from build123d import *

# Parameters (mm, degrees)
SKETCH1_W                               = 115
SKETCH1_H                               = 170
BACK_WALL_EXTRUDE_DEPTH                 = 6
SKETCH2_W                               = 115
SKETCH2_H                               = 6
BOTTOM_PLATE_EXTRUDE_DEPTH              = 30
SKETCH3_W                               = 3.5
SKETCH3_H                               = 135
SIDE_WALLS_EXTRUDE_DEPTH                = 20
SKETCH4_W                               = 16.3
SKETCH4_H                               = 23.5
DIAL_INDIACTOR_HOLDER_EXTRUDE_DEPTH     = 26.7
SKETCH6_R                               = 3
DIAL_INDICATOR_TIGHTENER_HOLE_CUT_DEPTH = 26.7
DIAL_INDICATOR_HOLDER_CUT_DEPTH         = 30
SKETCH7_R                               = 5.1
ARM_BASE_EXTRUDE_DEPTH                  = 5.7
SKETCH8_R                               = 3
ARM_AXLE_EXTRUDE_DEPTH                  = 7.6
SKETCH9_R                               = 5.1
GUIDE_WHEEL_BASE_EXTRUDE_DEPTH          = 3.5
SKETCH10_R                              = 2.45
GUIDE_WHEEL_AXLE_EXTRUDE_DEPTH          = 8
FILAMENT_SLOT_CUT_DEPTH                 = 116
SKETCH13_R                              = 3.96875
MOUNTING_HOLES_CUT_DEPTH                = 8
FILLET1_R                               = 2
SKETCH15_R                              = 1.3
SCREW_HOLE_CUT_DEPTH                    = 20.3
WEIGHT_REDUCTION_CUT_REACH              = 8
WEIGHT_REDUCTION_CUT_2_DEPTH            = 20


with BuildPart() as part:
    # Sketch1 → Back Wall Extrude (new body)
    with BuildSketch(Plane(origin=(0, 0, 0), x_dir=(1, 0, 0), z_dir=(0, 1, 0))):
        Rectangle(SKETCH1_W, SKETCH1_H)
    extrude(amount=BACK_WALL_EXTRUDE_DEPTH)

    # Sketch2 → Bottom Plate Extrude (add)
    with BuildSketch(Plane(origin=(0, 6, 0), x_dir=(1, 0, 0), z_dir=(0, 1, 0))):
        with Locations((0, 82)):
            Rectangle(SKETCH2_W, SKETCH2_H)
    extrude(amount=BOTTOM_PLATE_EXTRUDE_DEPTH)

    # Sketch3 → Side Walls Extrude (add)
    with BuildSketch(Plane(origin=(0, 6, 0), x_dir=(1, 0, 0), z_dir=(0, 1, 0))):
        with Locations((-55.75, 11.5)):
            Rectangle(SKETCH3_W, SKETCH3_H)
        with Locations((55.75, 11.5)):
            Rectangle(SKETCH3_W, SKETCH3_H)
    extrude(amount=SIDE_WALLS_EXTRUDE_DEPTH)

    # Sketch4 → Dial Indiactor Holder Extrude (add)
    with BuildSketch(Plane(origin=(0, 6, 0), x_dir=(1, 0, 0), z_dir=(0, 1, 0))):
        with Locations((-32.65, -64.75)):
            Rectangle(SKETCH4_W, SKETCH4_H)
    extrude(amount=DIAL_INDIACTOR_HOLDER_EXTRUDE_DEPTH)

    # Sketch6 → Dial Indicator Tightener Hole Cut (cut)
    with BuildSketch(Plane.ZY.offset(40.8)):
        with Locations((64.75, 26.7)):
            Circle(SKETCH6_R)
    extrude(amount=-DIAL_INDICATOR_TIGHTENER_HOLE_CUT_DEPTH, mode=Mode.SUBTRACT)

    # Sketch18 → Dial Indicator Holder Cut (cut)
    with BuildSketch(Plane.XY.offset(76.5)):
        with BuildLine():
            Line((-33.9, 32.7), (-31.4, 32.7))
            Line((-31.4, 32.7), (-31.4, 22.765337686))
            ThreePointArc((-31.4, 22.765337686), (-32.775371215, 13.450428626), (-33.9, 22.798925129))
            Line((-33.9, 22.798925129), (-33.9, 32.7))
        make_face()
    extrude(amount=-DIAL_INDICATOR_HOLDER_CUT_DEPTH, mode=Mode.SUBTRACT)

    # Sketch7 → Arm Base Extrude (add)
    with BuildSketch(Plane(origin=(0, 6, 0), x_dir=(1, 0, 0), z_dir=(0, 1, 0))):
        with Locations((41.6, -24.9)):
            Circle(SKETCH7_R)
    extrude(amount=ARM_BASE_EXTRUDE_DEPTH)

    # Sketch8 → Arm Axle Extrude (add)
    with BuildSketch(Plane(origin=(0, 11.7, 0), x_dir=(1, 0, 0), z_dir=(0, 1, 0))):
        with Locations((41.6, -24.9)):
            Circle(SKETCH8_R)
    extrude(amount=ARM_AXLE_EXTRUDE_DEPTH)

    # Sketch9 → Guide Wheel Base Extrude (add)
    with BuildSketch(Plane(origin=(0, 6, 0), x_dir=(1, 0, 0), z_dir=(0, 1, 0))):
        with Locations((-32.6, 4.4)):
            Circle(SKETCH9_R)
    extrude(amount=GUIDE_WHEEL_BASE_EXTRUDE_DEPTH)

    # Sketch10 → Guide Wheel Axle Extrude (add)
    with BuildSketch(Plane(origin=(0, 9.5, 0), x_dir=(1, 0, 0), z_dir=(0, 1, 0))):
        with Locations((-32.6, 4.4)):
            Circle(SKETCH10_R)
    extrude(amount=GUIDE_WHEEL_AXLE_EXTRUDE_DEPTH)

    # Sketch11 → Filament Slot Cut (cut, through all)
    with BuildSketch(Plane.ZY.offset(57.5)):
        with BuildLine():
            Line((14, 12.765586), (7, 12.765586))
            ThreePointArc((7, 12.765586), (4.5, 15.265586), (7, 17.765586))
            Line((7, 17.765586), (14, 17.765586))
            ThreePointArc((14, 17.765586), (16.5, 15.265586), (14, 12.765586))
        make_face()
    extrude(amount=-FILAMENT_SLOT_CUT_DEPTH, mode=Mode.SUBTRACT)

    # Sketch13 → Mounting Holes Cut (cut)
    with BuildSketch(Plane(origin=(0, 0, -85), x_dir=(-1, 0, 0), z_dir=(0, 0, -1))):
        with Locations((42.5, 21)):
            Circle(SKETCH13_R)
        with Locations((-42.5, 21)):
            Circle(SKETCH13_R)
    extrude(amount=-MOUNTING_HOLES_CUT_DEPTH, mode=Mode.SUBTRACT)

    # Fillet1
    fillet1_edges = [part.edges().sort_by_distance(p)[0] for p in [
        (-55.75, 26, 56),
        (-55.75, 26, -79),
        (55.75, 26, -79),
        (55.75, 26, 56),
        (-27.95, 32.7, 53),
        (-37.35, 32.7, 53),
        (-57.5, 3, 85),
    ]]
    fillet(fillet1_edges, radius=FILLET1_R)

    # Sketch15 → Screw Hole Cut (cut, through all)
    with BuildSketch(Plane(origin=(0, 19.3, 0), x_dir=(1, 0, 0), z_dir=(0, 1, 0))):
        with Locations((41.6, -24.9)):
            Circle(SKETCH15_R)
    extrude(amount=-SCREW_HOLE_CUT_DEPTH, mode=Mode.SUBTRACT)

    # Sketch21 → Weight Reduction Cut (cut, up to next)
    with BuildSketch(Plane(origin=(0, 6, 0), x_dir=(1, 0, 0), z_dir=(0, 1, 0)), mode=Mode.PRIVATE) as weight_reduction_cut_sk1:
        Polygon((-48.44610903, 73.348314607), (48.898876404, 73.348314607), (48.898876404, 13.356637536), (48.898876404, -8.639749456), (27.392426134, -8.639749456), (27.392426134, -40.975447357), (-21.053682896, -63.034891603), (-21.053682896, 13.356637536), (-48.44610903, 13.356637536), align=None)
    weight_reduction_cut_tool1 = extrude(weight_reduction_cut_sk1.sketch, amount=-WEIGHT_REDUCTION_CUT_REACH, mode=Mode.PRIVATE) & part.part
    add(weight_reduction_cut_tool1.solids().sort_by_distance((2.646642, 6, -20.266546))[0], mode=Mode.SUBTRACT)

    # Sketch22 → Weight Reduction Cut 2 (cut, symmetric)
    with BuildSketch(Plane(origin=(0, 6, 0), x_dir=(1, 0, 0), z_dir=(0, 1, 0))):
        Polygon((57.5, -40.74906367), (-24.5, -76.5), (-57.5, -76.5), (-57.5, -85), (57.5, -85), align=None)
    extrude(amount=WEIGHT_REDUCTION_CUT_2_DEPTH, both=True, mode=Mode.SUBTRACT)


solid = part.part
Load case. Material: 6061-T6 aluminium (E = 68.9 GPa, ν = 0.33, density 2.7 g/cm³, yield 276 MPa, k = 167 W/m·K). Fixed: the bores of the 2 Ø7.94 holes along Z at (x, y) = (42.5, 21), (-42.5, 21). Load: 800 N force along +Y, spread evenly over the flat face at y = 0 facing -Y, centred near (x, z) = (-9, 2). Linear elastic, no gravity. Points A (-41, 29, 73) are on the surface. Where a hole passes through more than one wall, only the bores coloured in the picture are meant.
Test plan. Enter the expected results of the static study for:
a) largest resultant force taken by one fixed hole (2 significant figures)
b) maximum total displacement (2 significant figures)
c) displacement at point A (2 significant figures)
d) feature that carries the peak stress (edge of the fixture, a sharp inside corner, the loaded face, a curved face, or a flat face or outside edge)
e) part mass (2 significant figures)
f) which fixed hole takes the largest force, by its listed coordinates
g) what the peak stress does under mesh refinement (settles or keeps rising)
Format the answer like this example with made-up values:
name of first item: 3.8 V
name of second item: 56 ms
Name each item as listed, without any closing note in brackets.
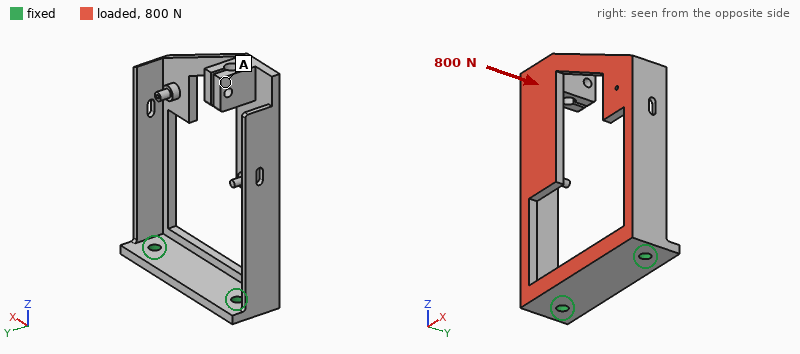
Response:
largest resultant force taken by one fixed hole: 540 N
maximum total displacement: 1.6 mm
displacement at point A: 1.5 mm
feature that carries the peak stress: a sharp inside corner
part mass: 250 g
which fixed hole takes the largest force, by its listed coordinates: (-42.5, 21)
what the peak stress does under mesh refinement: keeps rising
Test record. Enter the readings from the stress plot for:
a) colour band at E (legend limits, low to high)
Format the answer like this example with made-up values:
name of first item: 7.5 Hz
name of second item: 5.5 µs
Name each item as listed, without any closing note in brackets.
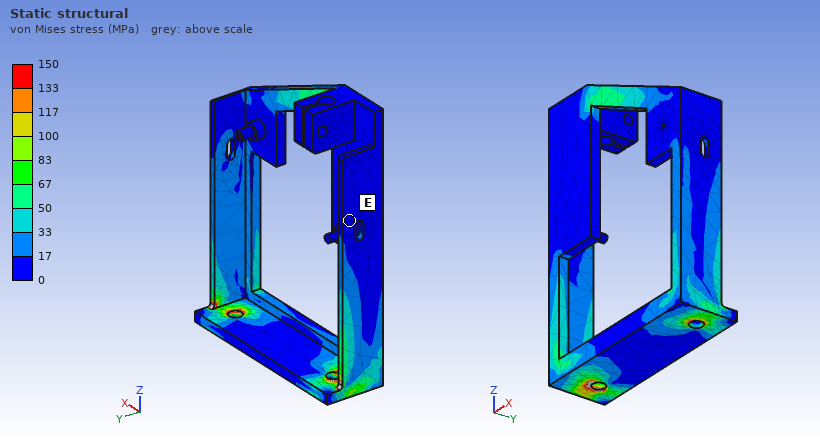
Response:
colour band at E: 0 to 17 MPa
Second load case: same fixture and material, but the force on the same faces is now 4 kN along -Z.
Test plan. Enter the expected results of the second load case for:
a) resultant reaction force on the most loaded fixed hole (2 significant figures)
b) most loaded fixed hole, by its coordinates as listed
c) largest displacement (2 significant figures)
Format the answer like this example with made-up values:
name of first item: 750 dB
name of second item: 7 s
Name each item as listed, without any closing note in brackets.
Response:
resultant reaction force on the most loaded fixed hole: 2.4 kN
most loaded fixed hole, by its coordinates as listed: (-42.5, 21)
largest displacement: 1.4 mm
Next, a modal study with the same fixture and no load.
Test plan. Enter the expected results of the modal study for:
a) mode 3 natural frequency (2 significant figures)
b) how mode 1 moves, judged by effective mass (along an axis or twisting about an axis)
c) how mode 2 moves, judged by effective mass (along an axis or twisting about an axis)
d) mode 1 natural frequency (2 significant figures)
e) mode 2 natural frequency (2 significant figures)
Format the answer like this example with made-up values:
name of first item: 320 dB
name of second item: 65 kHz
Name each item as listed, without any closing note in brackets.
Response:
mode 3 natural frequency: 680 Hz
how mode 1 moves, judged by effective mass: along Y
how mode 2 moves, judged by effective mass: along X
mode 1 natural frequency: 300 Hz
mode 2 natural frequency: 370 Hz
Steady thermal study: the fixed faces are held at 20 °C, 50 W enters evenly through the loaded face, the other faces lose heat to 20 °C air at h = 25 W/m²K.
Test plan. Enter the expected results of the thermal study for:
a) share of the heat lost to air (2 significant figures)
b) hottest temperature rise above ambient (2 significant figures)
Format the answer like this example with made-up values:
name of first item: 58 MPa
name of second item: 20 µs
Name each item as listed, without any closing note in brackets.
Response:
share of the heat lost to air: 46 %
hottest temperature rise above ambient: 49 K
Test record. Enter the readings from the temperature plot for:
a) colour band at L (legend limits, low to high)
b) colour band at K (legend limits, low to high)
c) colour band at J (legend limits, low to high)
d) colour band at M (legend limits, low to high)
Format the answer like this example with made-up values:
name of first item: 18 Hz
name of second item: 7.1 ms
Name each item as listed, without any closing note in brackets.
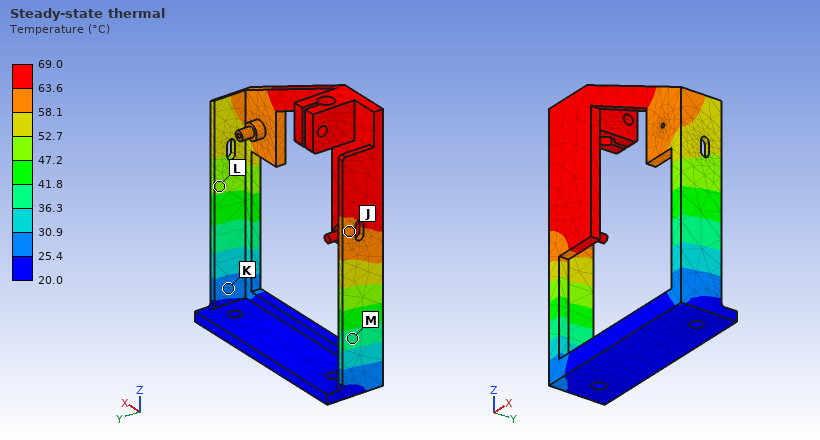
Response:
colour band at L: 47.2 to 52.7 °C
colour band at K: 25.4 to 30.9 °C
colour band at J: 58.1 to 63.6 °C
colour band at M: 36.3 to 41.8 °C
